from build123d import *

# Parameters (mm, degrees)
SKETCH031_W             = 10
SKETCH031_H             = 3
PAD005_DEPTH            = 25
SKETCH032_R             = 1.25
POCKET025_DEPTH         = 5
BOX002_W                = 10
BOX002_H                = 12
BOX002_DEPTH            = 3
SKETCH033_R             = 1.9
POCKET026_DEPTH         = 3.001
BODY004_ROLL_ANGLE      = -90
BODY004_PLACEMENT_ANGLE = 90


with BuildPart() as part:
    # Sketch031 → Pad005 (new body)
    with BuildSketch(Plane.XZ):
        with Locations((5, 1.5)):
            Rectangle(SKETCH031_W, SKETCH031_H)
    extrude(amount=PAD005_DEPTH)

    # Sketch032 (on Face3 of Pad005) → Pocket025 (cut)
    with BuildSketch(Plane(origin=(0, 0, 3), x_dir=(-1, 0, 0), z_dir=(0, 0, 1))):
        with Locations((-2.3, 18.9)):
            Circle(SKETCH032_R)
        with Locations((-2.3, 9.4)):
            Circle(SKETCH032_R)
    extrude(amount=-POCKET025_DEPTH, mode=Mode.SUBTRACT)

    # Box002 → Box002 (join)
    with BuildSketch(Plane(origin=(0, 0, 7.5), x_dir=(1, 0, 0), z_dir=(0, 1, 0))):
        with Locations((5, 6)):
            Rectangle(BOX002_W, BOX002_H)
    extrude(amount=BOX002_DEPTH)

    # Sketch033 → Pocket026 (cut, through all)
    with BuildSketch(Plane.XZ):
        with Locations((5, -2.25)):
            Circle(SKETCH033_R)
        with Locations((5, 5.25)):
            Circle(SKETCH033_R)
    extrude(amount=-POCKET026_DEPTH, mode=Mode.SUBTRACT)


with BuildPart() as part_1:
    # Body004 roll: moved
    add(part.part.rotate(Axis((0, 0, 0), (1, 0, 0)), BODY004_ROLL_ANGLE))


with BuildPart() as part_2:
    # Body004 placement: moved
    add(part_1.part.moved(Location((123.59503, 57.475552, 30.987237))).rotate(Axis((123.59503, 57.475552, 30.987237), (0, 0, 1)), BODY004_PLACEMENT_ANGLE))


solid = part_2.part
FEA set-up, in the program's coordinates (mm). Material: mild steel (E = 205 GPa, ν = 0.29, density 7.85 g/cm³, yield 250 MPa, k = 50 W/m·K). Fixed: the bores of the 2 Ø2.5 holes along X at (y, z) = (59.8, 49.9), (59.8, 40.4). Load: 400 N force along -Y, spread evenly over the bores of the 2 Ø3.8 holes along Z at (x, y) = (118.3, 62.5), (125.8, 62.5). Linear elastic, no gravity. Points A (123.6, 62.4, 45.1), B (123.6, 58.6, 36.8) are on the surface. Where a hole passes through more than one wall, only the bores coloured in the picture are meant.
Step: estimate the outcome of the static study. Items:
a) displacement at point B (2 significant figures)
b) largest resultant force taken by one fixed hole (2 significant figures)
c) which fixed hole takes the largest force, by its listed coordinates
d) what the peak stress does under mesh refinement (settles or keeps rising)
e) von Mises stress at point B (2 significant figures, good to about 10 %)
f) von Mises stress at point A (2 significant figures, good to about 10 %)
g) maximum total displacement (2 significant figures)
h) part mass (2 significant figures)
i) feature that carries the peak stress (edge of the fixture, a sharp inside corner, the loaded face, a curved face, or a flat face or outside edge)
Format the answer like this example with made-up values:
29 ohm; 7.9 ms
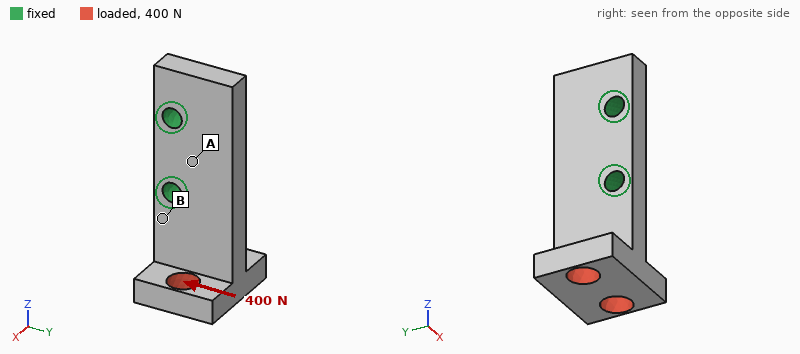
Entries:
2.3 µm; 730 N; (59.8, 40.4); keeps rising; 50 MPa; 27 MPa; 11 µm; 7.9 g; edge of the fixture
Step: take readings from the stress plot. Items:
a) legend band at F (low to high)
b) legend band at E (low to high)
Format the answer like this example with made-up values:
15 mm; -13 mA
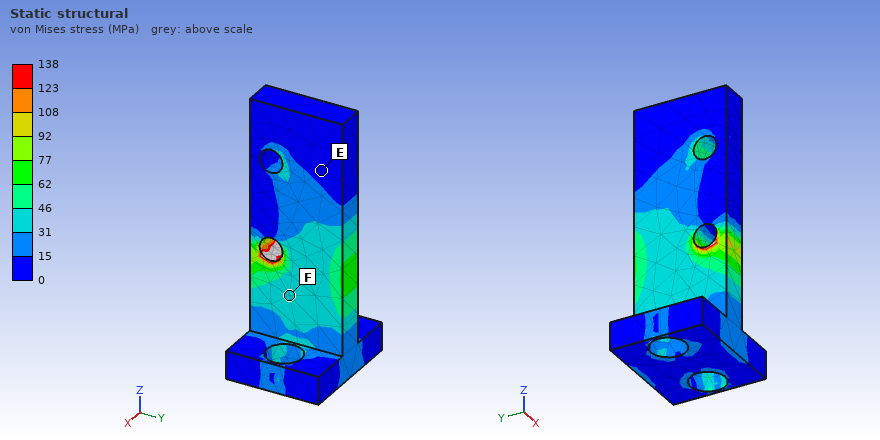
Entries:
31 to 46 MPa; 0 to 15 MPa
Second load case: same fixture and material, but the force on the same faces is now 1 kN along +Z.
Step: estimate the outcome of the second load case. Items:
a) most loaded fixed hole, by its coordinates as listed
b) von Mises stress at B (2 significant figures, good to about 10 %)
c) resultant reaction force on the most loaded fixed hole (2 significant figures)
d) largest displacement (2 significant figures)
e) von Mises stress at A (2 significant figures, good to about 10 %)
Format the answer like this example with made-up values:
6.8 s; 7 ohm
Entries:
(59.8, 40.4); 33 MPa; 800 N; 9.5 µm; 21 MPa
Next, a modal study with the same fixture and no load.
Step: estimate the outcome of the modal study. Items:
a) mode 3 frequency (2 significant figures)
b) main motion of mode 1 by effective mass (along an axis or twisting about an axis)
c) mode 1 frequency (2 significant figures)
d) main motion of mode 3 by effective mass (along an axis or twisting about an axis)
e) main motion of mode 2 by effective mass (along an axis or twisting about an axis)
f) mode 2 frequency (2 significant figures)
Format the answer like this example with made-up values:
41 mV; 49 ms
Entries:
20 kHz; along X; 8800 Hz; along Y; twisting about Z; 17 kHz
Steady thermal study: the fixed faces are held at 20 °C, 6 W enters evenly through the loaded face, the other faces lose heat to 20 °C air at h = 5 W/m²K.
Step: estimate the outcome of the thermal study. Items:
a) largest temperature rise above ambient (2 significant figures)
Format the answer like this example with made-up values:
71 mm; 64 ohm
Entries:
56 K
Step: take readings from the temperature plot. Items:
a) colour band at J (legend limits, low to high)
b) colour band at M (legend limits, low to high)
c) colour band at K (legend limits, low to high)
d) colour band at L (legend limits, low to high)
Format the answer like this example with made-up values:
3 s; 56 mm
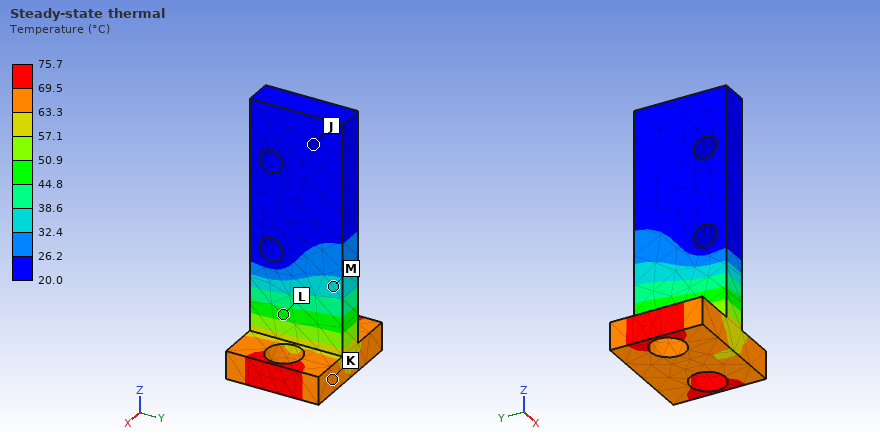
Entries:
20.0 to 26.2 °C; 32.4 to 38.6 °C; 63.3 to 69.5 °C; 44.8 to 50.9 °C
